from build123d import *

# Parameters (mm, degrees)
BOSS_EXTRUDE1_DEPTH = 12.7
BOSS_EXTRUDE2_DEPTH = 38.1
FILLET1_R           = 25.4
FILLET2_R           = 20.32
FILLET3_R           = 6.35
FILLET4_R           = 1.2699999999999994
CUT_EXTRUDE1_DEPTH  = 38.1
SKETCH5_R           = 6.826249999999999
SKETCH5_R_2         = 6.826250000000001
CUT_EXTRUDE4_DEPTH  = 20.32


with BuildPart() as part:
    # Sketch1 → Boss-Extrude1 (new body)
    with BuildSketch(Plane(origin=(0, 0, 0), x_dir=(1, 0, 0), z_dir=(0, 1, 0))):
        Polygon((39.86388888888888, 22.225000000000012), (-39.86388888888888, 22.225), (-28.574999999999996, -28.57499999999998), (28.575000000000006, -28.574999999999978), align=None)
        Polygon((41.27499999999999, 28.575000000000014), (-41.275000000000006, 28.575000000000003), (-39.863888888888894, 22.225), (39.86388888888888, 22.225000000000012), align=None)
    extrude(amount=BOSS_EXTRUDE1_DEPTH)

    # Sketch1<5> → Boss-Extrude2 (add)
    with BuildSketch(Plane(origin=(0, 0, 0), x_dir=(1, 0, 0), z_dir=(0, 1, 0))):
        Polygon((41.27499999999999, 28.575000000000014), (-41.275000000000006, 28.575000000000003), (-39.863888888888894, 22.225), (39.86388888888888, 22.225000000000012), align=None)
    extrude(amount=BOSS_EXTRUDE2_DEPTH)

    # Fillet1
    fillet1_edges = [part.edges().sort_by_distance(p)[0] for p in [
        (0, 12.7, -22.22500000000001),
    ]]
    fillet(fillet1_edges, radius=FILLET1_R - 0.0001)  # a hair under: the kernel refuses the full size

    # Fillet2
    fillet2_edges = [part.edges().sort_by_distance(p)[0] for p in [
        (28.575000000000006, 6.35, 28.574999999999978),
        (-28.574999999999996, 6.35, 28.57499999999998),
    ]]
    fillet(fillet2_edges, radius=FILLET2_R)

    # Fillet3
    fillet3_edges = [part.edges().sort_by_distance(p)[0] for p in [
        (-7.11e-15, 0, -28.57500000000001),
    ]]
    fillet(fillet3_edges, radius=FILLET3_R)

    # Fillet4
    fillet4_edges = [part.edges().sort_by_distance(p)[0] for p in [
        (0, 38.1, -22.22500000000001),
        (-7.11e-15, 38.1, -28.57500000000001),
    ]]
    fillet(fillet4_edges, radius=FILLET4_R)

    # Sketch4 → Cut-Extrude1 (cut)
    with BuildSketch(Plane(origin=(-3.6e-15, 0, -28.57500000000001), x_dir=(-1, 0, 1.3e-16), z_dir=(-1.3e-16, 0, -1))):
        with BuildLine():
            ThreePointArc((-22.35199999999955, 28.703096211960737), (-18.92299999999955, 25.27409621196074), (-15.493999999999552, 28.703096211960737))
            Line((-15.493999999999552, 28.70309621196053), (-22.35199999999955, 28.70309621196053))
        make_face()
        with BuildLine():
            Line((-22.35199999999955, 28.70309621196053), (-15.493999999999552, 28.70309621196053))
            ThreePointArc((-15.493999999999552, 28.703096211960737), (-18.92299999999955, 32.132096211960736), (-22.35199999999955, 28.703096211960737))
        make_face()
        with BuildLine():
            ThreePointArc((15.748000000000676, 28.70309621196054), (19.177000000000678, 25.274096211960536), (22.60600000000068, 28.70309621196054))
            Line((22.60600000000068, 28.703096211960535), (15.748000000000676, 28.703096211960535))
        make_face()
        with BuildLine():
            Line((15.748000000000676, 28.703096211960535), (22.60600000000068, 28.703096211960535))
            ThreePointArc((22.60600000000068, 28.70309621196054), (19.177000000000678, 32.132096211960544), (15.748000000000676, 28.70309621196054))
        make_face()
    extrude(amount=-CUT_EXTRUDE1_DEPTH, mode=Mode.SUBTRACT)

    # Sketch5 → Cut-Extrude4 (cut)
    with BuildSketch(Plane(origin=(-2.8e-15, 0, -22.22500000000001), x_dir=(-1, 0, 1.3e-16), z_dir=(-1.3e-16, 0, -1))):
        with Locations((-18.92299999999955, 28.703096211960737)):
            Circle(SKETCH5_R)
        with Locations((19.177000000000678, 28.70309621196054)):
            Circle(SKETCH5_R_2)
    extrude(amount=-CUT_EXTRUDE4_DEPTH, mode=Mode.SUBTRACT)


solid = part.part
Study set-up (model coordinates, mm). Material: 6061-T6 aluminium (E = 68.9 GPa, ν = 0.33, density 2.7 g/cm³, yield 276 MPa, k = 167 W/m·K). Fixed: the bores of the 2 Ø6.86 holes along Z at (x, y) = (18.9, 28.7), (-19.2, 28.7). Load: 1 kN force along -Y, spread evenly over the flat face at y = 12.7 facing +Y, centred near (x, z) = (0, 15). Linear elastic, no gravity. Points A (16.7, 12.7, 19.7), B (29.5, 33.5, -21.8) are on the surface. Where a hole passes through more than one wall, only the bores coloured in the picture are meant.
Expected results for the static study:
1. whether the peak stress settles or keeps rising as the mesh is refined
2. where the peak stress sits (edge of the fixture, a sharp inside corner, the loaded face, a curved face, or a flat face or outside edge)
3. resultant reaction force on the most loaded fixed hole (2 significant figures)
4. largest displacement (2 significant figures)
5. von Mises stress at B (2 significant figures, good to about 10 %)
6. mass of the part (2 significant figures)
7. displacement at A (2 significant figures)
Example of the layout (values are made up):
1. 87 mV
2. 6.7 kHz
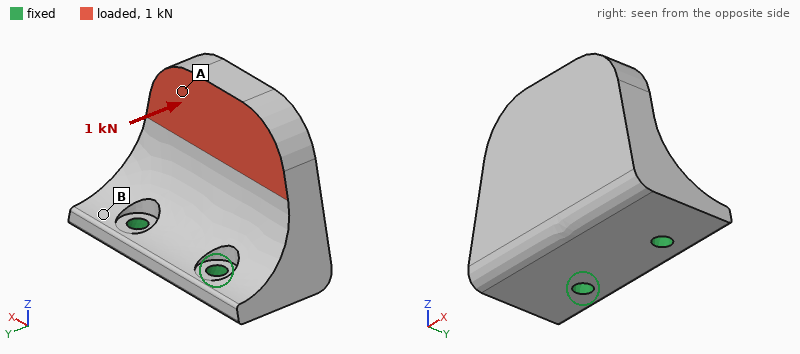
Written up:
1. keeps rising
2. edge of the fixture
3. 520 N
4. 0.16 mm
5. 25 MPa
6. 190 g
7. 0.12 mm
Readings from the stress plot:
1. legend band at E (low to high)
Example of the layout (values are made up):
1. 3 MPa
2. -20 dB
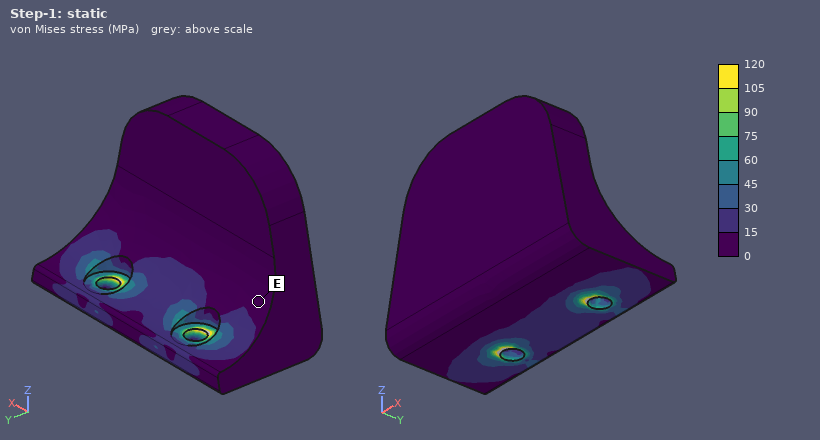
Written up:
1. 0 to 15 MPa
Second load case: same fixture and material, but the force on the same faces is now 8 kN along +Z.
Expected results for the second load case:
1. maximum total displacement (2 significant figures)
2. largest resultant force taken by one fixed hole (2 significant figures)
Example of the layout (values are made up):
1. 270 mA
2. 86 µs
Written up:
1. 0.32 mm
2. 4.0 kN
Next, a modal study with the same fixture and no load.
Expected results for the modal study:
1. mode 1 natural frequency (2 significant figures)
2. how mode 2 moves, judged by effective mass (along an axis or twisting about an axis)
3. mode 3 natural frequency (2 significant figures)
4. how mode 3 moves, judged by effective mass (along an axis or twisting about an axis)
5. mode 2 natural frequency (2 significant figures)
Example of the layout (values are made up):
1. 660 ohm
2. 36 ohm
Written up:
1. 1600 Hz
2. along X
3. 7300 Hz
4. along X
5. 4100 Hz
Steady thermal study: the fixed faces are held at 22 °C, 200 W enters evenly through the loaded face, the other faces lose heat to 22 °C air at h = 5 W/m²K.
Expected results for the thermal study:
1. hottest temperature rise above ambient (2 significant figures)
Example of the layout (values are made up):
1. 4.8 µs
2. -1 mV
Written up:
1. 81 K
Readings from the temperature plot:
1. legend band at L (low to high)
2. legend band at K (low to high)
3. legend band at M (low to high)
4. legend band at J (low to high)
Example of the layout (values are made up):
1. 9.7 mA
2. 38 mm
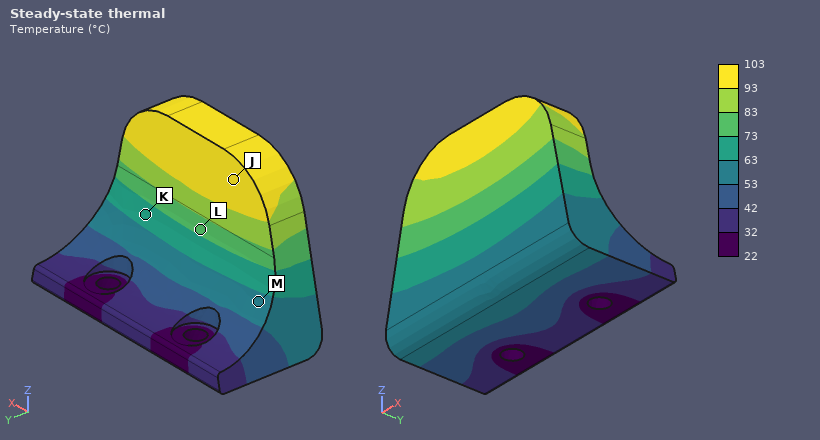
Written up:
1. 73 to 83 °C
2. 63 to 73 °C
3. 53 to 63 °C
4. 93 to 103 °C
